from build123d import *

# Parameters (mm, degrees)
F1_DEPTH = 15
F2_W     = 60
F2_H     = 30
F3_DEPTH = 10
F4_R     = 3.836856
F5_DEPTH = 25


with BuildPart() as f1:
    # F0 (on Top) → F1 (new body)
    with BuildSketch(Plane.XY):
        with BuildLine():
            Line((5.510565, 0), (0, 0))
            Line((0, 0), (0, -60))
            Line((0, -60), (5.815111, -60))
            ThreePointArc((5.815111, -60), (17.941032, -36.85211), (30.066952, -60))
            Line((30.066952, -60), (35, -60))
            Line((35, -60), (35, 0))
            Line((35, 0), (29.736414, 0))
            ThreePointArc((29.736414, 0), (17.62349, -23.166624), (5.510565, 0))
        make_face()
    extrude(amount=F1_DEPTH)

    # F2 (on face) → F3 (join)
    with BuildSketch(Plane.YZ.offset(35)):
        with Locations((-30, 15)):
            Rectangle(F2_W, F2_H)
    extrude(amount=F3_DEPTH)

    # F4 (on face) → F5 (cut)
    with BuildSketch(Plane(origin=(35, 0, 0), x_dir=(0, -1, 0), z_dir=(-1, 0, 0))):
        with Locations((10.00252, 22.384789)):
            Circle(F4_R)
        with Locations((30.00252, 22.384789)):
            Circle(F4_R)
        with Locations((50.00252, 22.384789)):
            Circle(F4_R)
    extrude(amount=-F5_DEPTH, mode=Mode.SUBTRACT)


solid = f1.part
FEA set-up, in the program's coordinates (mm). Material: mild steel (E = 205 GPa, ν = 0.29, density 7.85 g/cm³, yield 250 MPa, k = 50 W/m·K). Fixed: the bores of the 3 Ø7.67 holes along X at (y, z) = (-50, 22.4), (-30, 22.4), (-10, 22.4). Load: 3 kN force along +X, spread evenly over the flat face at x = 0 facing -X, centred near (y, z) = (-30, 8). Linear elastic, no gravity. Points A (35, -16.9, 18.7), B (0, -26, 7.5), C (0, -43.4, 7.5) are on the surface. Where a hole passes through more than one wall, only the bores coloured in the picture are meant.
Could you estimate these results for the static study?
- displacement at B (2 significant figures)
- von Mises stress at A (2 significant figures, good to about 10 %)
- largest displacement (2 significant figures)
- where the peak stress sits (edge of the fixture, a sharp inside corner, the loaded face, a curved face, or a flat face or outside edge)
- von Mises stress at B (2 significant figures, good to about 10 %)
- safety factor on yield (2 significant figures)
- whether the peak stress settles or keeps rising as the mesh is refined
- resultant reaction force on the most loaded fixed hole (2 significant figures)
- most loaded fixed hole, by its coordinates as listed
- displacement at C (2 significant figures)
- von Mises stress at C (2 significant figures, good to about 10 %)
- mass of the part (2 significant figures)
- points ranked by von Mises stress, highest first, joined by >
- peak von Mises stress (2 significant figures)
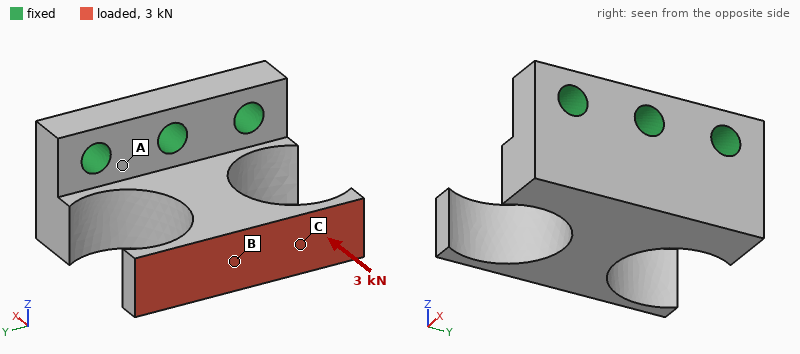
13 µm
20 MPa
69 µm
a curved face
47 MPa
1.8
settles
1.5 kN
(-30, 22.4)
16 µm
94 MPa
240 g
C > B > A
140 MPa
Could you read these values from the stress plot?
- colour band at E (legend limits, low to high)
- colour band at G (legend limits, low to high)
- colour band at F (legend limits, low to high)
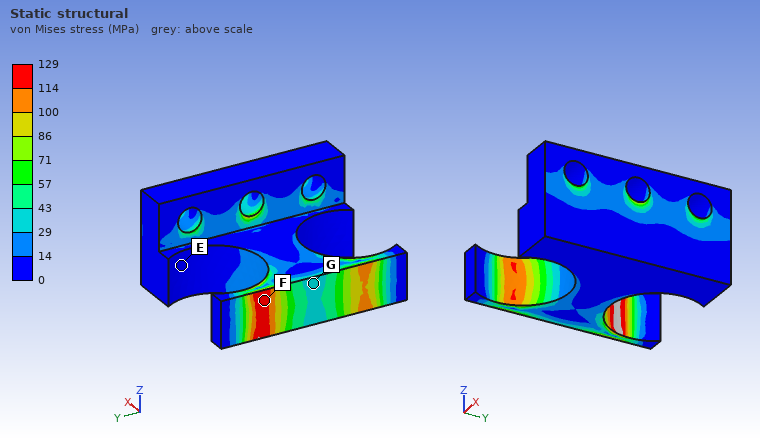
0 to 14 MPa
29 to 43 MPa
114 to 129 MPa
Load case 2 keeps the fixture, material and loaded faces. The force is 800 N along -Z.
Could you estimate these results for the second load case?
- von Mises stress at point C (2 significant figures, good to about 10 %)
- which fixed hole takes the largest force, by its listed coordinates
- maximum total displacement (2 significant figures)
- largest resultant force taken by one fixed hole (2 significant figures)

8.9 MPa
(-30, 22.4)
33 µm
650 N
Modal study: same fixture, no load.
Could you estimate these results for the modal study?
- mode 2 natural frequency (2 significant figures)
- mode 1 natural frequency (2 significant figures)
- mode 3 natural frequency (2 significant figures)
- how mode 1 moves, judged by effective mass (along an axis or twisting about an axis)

5300 Hz
3900 Hz
7300 Hz
along Z
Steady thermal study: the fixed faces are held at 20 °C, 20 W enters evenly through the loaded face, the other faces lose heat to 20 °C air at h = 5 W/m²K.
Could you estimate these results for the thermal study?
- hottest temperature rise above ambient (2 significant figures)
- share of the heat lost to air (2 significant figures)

82 K
4.2 %
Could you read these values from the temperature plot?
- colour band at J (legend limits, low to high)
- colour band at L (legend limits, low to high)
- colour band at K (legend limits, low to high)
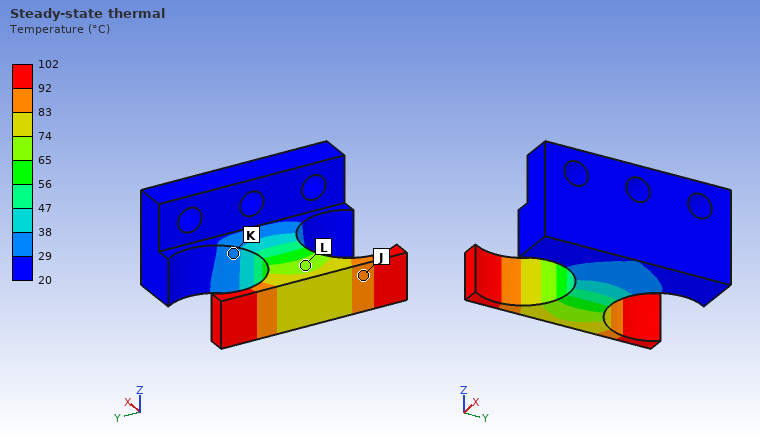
83 to 92 °C
65 to 74 °C
29 to 38 °C
